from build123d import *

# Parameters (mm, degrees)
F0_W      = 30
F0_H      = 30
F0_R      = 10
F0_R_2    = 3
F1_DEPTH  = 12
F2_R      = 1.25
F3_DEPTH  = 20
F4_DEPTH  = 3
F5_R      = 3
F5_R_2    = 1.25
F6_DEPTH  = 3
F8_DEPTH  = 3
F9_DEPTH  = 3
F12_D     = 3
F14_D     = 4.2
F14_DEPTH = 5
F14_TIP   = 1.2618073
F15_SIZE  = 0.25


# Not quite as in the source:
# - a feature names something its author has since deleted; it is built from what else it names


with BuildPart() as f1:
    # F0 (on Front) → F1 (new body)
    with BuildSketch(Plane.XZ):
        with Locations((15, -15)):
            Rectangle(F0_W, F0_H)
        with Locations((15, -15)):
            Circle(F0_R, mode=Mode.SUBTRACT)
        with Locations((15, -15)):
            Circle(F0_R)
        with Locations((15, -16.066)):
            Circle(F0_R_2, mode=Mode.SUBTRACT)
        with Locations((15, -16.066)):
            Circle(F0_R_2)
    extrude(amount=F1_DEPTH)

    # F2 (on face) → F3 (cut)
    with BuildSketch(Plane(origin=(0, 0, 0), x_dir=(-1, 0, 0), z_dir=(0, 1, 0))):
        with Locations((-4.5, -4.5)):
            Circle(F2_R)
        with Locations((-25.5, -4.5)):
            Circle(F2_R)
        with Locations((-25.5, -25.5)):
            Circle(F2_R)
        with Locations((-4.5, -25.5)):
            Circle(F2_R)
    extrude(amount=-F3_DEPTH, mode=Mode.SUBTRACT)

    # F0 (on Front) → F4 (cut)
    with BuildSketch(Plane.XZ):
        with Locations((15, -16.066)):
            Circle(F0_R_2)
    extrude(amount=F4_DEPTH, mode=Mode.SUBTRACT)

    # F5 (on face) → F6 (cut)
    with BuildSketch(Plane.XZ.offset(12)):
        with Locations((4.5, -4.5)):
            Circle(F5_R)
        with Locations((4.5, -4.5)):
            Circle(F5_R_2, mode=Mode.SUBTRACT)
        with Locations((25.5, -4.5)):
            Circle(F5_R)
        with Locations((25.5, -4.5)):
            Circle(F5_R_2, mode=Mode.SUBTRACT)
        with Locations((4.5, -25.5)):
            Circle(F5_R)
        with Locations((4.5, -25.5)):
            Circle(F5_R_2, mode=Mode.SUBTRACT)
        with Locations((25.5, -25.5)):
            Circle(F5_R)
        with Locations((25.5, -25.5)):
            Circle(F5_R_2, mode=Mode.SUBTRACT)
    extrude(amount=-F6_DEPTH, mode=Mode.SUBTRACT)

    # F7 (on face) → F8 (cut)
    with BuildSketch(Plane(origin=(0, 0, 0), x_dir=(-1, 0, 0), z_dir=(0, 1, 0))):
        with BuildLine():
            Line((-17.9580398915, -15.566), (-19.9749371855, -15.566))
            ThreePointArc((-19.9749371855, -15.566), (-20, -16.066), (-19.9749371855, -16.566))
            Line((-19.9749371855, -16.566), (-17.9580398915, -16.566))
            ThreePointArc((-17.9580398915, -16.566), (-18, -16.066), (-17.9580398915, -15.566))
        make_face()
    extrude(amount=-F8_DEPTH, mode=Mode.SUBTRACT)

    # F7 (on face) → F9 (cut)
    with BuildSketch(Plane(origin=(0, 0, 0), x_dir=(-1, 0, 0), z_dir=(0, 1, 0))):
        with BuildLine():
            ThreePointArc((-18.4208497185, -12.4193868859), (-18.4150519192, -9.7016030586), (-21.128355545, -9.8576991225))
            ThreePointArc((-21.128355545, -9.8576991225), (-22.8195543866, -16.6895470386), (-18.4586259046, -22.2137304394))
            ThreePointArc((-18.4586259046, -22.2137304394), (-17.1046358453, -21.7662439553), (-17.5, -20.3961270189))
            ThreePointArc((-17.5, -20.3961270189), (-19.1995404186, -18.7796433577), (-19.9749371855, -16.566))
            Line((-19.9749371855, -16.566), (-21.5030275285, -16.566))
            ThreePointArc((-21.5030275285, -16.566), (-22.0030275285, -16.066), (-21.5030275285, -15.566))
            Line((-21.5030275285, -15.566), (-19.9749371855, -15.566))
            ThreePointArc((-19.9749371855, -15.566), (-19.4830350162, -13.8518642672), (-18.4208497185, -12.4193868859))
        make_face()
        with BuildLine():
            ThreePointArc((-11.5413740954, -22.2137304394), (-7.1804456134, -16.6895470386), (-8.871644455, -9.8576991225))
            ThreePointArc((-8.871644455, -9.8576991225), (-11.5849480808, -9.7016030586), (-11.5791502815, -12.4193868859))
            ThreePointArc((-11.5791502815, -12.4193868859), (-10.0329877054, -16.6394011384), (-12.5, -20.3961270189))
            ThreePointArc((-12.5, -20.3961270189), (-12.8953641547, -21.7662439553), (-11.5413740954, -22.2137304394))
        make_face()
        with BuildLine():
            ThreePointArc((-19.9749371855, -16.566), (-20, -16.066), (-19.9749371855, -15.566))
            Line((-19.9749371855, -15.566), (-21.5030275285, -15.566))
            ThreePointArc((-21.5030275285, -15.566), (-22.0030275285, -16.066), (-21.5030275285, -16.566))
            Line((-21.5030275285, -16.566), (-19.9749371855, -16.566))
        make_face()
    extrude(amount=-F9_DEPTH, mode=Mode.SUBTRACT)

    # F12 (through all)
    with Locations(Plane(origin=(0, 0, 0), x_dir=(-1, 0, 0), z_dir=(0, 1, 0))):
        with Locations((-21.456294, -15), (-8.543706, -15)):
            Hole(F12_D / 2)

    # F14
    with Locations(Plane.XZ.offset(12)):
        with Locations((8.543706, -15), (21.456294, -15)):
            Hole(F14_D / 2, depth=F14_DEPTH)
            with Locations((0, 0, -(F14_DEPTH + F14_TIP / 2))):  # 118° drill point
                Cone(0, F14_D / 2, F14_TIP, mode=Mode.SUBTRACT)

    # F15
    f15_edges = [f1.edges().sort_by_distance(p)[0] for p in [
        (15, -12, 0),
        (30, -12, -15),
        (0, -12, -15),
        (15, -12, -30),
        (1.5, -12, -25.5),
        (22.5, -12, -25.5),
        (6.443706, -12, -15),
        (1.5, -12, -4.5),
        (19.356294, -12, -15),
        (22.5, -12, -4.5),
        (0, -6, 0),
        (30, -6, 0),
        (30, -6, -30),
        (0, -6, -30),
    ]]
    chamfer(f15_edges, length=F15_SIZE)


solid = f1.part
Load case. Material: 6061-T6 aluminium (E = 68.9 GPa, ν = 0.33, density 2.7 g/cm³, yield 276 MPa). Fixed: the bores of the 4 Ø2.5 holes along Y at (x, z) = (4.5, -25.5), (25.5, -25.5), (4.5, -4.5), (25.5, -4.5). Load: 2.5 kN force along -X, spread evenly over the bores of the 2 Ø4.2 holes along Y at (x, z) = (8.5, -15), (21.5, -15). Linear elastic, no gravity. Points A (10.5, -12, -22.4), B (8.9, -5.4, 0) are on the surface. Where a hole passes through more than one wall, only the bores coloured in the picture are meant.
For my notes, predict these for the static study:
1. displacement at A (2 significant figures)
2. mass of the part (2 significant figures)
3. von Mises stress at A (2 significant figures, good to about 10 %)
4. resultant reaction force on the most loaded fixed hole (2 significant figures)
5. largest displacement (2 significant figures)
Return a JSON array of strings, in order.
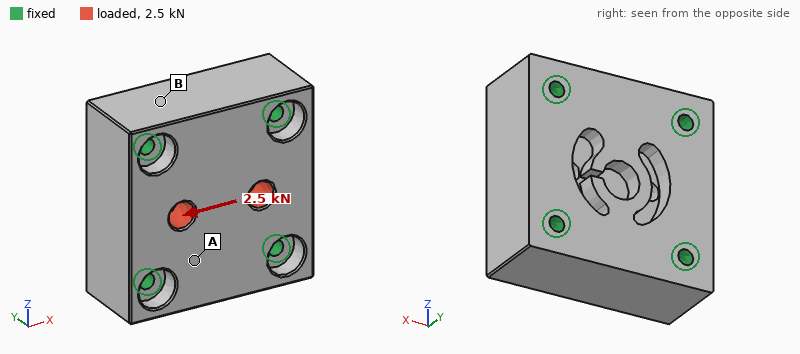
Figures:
["1.4 µm", "26 g", "7.6 MPa", "710 N", "3.4 µm"]
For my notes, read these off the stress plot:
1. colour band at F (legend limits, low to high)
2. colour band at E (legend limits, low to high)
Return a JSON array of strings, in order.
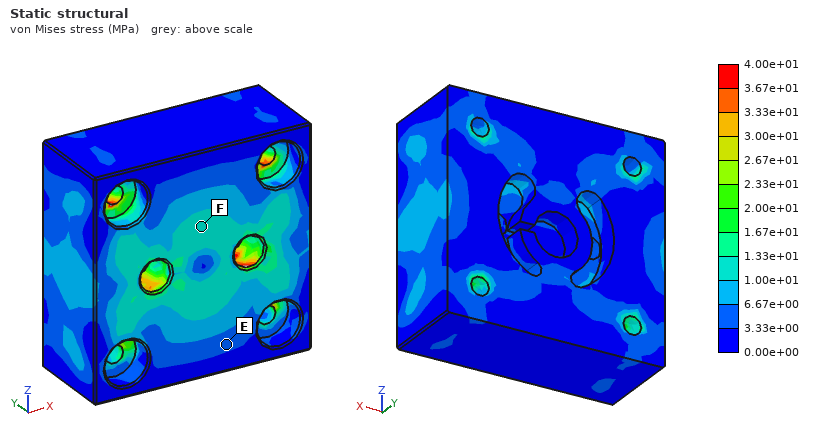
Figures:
["1.00e+01 to 1.33e+01 MPa", "3.33e+00 to 6.67e+00 MPa"]
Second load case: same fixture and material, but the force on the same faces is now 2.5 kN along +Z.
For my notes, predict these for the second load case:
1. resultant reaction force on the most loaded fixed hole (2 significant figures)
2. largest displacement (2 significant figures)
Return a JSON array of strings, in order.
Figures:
["690 N", "2.5 µm"]
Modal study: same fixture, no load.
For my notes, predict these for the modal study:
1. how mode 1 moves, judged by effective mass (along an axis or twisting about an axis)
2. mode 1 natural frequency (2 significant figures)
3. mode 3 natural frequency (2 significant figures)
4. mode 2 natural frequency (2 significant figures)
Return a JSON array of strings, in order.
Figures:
["along Y", "43 kHz", "55 kHz", "53 kHz"]
